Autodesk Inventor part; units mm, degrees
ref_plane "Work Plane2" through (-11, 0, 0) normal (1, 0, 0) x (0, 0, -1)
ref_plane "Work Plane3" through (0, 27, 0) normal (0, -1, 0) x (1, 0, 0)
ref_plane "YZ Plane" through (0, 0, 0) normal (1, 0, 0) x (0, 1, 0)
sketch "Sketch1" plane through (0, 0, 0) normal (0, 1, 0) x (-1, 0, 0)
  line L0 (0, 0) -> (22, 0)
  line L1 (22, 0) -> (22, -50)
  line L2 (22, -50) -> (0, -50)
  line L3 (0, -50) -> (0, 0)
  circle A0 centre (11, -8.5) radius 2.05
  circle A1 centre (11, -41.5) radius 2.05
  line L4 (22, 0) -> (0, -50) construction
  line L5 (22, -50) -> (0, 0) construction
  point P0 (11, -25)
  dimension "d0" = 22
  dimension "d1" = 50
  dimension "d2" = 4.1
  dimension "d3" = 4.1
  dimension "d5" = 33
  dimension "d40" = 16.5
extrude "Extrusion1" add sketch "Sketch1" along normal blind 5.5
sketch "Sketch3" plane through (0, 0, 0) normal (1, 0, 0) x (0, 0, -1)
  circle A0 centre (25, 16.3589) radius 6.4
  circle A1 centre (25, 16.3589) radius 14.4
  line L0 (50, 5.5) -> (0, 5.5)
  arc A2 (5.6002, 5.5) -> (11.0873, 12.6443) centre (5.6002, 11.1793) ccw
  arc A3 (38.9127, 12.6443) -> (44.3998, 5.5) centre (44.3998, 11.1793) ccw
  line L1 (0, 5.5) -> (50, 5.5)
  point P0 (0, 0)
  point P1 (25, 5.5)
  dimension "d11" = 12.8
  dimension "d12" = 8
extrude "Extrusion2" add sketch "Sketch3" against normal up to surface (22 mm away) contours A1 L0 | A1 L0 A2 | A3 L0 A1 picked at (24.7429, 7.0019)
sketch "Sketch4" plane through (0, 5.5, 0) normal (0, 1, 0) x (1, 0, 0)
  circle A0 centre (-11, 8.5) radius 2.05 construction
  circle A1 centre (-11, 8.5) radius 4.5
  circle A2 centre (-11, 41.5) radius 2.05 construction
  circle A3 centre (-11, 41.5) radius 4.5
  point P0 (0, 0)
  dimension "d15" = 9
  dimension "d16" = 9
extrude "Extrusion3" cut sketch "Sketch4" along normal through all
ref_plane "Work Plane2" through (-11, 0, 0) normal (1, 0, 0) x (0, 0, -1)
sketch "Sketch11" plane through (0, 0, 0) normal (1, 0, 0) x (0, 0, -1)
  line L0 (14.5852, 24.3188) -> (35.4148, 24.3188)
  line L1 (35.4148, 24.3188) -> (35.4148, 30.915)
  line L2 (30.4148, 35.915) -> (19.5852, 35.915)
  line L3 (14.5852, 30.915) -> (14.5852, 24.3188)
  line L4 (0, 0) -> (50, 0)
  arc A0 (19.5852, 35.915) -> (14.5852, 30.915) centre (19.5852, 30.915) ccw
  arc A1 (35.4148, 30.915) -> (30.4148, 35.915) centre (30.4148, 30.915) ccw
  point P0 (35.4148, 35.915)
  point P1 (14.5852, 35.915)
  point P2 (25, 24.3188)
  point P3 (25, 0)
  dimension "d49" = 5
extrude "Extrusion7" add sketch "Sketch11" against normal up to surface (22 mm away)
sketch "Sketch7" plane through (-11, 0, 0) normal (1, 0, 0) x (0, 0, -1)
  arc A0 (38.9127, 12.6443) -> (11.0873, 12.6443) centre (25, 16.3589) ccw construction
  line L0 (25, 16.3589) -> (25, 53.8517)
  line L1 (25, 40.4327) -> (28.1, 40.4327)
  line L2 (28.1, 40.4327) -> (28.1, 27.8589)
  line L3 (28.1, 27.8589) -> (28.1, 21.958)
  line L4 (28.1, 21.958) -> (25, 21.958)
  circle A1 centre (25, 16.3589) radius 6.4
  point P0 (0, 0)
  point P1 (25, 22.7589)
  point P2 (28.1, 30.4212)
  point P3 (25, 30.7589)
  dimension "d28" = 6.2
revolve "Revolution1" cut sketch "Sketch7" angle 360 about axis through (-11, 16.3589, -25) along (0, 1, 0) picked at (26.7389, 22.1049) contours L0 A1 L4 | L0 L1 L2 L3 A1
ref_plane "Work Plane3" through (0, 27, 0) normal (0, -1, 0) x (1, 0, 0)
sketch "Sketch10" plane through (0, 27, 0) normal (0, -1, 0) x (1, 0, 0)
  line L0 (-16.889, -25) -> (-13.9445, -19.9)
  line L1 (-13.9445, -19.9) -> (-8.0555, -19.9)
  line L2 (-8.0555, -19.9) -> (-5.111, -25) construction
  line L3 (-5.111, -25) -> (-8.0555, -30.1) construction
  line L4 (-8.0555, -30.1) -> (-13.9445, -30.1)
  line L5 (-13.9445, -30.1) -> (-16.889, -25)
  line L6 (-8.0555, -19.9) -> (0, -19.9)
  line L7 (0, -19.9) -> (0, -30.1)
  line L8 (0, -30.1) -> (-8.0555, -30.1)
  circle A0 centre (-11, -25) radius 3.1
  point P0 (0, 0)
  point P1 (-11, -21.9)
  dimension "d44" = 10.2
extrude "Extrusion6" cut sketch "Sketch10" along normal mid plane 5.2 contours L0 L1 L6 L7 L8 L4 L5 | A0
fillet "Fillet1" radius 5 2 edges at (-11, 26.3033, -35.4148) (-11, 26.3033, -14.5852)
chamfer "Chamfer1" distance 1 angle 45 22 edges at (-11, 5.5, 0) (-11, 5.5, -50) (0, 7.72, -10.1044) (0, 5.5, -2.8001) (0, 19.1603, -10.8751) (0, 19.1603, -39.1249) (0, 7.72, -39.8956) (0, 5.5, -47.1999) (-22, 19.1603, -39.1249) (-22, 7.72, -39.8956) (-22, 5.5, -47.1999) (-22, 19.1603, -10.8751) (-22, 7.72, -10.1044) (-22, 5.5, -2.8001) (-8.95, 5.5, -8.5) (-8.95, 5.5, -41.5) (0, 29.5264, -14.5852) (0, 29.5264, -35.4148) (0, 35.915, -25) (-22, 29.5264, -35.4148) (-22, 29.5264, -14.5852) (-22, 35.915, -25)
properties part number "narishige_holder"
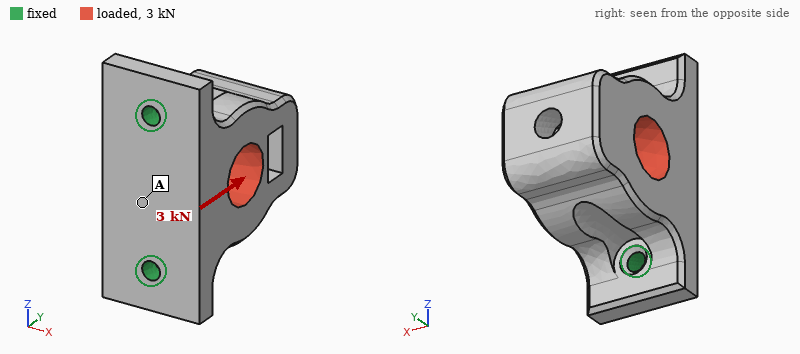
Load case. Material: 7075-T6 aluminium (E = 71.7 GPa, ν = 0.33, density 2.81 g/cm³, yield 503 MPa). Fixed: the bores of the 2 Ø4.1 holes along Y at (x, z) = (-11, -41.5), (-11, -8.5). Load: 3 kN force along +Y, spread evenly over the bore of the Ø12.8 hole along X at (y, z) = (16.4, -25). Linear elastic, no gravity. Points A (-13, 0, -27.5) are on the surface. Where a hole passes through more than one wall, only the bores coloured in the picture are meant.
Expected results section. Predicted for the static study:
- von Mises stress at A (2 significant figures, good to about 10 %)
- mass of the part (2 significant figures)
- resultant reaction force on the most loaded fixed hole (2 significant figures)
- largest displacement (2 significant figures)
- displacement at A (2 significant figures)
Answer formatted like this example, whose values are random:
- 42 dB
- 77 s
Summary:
- 9.9 MPa
- 51 g
- 1.7 kN
- 8.9 µm
- 7.2 µm
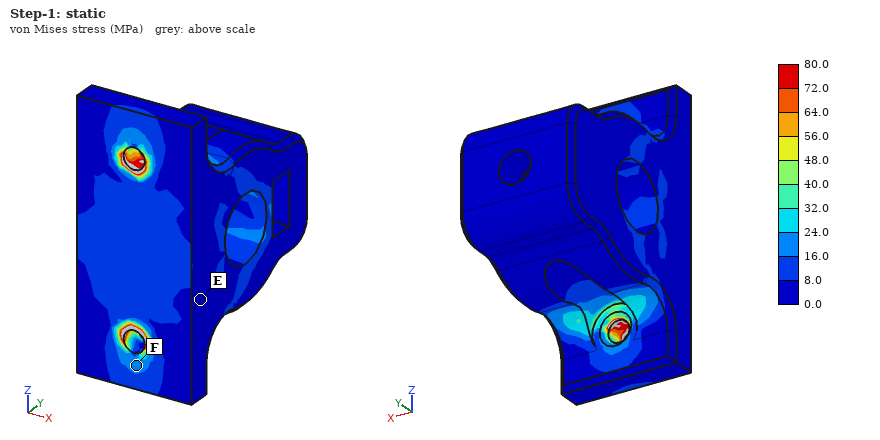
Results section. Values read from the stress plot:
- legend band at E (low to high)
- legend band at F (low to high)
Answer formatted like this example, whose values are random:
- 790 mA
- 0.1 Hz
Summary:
- 0.0 to 8.0 MPa
- 16.0 to 24.0 MPa
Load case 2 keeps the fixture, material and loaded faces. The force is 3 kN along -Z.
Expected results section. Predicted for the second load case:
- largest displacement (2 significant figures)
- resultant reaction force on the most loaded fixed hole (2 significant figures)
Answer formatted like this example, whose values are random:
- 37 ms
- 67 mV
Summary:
- 19 µm
- 2.0 kN
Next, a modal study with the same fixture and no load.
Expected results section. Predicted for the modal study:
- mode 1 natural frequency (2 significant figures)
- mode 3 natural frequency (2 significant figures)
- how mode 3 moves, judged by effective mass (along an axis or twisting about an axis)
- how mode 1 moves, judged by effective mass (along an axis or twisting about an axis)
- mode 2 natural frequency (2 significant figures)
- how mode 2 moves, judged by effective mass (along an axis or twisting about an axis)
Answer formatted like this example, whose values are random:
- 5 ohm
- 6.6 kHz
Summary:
- 4000 Hz
- 16 kHz
- along Y
- along X
- 10 kHz
- along Z
